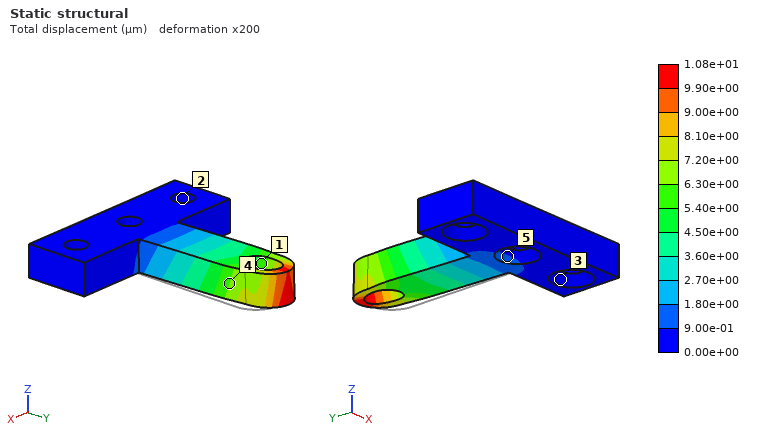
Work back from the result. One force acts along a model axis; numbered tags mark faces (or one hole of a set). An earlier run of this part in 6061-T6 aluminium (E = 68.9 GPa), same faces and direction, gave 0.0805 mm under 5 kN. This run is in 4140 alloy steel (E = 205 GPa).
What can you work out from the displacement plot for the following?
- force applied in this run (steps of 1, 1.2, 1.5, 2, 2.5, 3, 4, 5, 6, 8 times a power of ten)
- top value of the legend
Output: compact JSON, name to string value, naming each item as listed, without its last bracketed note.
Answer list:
{"force applied in this run": "2 kN", "top value of the legend": "1.08e+01 µm"}
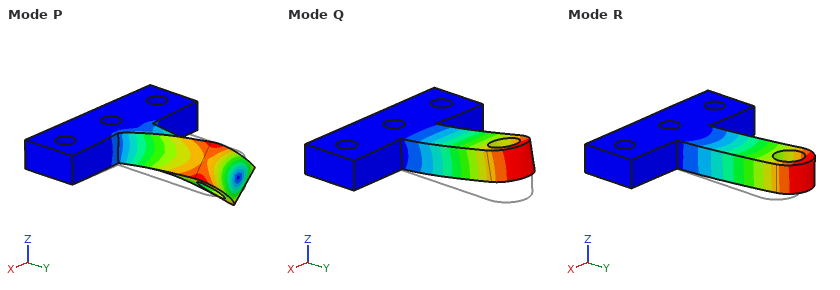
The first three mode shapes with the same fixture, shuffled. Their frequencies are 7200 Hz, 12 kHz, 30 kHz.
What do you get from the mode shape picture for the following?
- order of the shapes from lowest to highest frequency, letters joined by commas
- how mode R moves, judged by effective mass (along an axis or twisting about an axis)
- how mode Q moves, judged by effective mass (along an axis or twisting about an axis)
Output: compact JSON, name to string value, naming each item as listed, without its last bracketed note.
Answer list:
{"order of the shapes from lowest to highest frequency, letters joined by commas": "Q, R, P", "how mode R moves, judged by effective mass": "along X", "how mode Q moves, judged by effective mass": "along Z"}
